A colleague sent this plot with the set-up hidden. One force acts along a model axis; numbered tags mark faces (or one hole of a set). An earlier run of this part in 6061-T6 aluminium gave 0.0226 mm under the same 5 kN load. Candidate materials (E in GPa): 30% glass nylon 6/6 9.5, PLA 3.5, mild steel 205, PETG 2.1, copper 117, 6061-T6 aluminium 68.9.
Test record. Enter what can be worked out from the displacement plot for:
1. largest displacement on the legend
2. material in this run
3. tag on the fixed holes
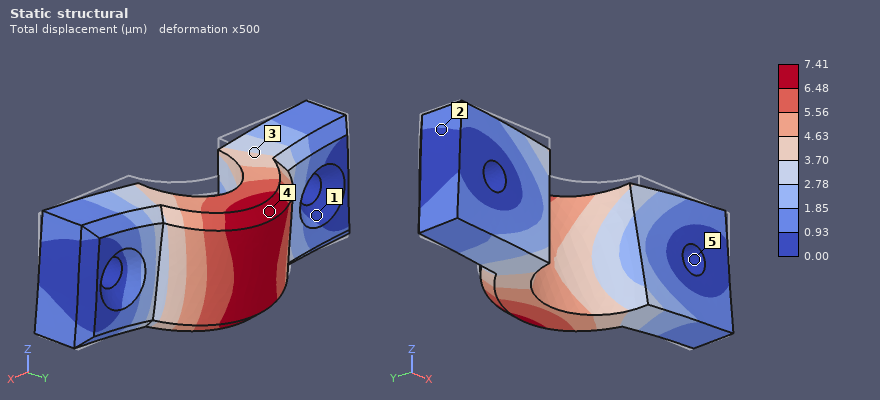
7.41 µm
mild steel
5
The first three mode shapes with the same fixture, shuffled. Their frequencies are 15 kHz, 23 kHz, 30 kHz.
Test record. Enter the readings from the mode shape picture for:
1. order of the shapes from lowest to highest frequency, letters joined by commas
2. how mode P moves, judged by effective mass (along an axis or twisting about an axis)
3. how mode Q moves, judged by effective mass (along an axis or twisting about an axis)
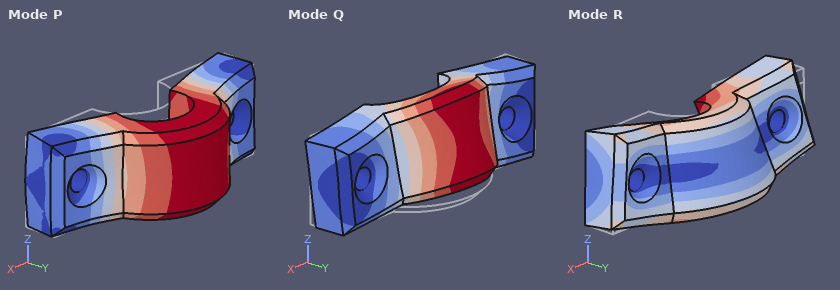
Q, P, R
along Y
along Z
